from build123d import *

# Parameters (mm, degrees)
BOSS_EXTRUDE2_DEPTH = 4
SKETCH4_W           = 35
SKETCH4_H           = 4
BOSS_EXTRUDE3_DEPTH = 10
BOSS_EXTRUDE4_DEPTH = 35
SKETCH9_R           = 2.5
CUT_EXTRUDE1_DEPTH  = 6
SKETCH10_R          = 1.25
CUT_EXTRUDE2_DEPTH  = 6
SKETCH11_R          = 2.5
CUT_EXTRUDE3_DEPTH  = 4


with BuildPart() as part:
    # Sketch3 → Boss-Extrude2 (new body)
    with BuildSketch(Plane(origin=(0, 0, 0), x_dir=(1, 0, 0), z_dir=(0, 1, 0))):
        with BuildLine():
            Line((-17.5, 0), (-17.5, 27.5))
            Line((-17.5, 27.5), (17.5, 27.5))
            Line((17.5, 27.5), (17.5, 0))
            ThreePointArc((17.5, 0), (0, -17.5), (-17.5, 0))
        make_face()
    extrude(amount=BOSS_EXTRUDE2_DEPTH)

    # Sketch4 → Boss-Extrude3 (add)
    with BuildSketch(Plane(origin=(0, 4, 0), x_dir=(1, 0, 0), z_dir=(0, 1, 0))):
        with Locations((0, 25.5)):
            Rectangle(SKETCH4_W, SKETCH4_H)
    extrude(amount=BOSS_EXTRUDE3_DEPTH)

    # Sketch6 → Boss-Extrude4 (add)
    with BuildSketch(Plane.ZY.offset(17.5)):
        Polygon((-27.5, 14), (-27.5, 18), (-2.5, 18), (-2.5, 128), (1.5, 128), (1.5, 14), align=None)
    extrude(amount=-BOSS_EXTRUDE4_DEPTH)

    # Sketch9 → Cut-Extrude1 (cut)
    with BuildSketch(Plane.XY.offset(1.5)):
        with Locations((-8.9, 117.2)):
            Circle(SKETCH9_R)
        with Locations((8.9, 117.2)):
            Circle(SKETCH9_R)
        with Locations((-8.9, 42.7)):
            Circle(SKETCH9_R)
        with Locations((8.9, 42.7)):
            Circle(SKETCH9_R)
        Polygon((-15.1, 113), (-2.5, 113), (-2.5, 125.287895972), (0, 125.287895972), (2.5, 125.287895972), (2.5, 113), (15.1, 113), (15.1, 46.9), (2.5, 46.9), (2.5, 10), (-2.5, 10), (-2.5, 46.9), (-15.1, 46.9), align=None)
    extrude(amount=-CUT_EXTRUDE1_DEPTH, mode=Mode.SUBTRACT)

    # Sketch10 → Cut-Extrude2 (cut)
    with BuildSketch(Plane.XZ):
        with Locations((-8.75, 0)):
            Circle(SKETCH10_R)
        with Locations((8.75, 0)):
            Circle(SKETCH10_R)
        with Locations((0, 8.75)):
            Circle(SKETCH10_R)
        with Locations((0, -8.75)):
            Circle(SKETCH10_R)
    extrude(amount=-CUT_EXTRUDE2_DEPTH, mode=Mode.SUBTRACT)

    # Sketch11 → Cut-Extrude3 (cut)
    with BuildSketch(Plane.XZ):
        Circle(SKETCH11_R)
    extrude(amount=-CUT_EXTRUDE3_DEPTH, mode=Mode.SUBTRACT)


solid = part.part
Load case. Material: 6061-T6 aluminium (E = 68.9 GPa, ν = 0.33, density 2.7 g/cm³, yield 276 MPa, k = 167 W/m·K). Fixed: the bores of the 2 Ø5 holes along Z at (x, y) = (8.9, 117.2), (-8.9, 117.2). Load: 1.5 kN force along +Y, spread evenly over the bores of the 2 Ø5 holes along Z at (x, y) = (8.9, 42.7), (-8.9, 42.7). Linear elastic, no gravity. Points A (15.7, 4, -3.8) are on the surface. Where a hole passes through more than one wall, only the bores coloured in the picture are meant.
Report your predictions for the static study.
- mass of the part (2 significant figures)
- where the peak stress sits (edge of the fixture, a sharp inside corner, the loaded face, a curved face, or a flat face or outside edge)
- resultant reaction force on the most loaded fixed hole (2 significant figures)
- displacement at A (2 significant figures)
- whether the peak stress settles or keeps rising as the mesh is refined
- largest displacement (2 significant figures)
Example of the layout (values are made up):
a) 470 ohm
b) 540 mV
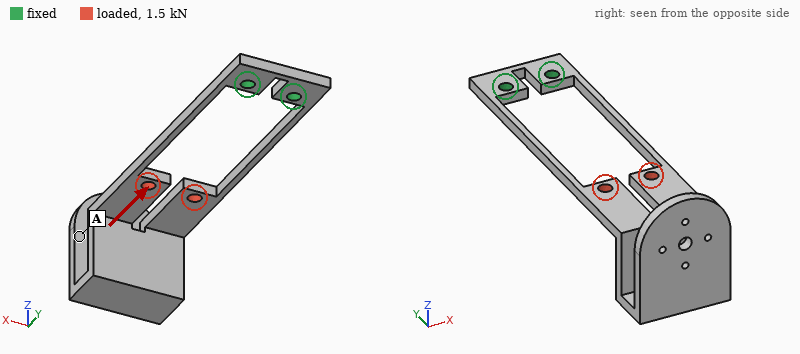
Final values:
a) 47 g
b) a sharp inside corner
c) 790 N
d) 0.15 mm
e) keeps rising
f) 0.36 mm
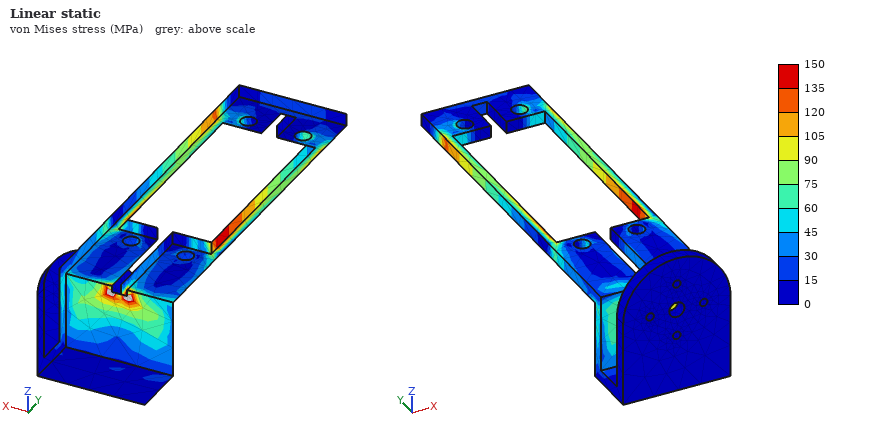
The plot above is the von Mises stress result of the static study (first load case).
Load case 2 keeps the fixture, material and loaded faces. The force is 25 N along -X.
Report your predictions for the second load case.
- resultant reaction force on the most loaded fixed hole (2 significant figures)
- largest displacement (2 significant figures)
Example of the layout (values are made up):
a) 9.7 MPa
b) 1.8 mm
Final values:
a) 39 N
b) 1.1 mm
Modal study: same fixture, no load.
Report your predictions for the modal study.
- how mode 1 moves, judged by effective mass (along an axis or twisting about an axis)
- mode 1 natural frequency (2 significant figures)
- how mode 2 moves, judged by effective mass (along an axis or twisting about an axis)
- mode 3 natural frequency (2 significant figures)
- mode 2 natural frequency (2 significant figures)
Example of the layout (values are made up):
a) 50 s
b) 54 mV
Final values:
a) along Z
b) 55 Hz
c) along X
d) 240 Hz
e) 110 Hz
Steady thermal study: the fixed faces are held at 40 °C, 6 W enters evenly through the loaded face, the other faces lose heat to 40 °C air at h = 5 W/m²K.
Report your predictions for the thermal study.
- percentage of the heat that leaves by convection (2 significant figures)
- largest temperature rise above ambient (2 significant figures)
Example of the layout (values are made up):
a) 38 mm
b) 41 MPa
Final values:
a) 51 %
b) 70 K
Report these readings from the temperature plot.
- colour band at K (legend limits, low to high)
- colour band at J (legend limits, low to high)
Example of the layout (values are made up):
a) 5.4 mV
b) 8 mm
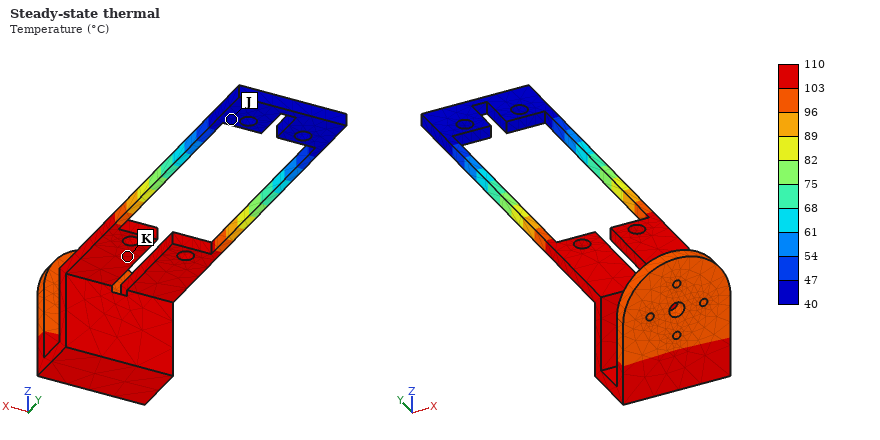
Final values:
a) 103 to 110 °C
b) 40 to 47 °C
